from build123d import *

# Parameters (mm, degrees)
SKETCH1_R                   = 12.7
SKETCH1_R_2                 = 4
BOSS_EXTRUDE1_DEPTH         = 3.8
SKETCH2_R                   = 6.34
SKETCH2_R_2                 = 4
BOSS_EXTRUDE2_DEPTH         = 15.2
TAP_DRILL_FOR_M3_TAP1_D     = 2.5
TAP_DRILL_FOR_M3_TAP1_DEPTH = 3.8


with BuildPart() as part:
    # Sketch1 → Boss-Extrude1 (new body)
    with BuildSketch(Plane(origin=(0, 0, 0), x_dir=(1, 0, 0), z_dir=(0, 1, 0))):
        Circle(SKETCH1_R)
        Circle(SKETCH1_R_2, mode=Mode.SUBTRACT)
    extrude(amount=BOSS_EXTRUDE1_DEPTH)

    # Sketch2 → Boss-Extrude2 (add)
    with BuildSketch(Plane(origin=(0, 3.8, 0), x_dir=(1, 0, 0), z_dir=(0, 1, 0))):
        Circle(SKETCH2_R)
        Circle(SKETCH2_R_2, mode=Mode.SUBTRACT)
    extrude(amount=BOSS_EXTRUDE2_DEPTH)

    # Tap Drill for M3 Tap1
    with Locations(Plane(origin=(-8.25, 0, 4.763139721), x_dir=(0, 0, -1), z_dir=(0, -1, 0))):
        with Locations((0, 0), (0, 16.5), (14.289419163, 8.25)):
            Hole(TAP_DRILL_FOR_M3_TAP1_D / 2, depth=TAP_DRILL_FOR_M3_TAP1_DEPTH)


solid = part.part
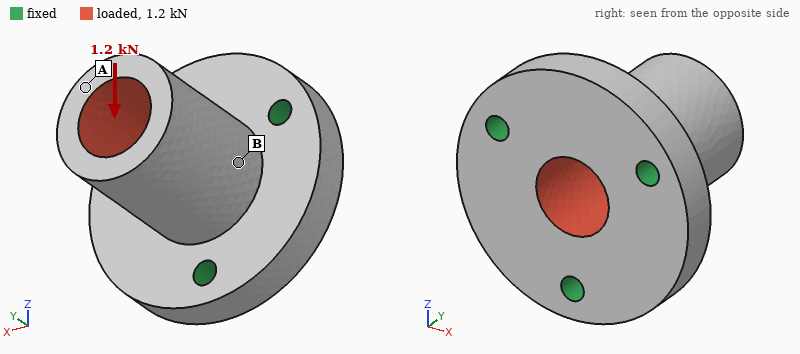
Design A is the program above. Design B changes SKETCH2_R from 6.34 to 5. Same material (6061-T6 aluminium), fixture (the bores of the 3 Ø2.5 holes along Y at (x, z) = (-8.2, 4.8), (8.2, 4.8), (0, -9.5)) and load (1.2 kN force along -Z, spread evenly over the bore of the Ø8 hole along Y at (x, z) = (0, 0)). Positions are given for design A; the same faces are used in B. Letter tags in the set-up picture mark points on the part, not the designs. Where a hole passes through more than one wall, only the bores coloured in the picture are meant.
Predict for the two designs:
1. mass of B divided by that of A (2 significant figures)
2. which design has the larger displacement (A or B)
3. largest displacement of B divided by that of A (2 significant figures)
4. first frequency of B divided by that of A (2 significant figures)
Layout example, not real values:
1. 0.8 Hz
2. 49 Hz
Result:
1. 0.74
2. B
3. 2.6
4. 1.0
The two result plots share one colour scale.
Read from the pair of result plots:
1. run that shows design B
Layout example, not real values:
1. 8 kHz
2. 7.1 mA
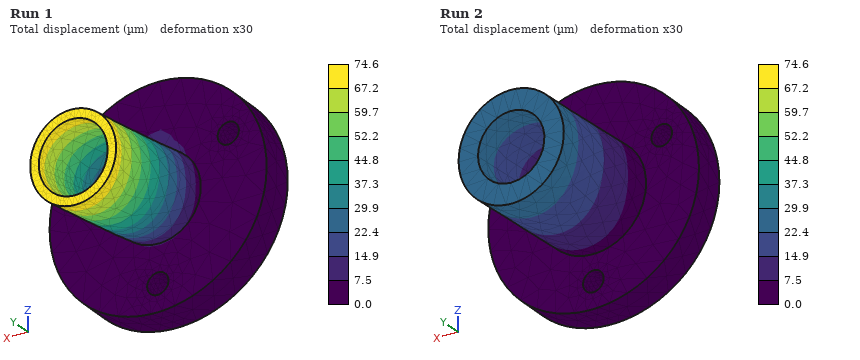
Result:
1. Run 1
